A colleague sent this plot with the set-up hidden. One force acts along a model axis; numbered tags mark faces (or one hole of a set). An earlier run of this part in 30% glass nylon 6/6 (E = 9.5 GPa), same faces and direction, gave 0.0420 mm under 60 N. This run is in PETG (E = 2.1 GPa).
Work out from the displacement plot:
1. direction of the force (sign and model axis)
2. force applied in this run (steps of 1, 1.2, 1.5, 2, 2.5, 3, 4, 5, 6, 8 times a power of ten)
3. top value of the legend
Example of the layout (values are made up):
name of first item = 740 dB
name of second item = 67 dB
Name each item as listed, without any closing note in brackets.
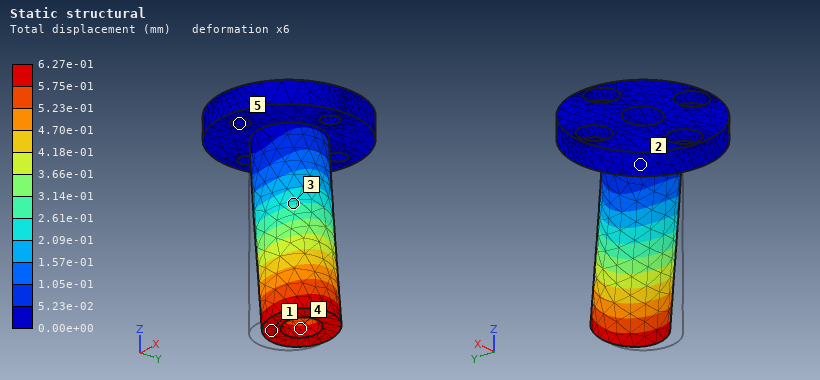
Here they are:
direction of the force = +X
force applied in this run = 200 N
top value of the legend = 6.27e-01 mm
